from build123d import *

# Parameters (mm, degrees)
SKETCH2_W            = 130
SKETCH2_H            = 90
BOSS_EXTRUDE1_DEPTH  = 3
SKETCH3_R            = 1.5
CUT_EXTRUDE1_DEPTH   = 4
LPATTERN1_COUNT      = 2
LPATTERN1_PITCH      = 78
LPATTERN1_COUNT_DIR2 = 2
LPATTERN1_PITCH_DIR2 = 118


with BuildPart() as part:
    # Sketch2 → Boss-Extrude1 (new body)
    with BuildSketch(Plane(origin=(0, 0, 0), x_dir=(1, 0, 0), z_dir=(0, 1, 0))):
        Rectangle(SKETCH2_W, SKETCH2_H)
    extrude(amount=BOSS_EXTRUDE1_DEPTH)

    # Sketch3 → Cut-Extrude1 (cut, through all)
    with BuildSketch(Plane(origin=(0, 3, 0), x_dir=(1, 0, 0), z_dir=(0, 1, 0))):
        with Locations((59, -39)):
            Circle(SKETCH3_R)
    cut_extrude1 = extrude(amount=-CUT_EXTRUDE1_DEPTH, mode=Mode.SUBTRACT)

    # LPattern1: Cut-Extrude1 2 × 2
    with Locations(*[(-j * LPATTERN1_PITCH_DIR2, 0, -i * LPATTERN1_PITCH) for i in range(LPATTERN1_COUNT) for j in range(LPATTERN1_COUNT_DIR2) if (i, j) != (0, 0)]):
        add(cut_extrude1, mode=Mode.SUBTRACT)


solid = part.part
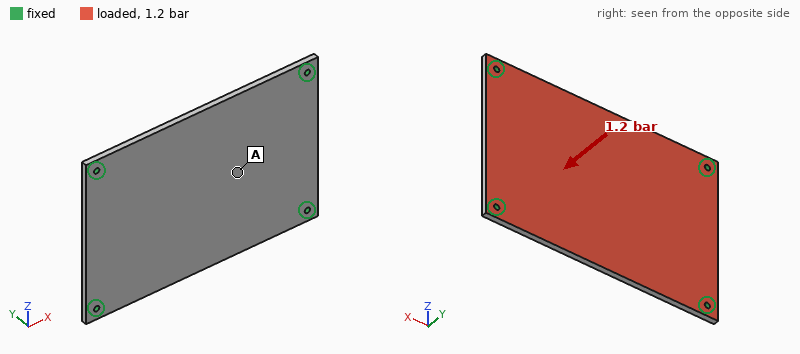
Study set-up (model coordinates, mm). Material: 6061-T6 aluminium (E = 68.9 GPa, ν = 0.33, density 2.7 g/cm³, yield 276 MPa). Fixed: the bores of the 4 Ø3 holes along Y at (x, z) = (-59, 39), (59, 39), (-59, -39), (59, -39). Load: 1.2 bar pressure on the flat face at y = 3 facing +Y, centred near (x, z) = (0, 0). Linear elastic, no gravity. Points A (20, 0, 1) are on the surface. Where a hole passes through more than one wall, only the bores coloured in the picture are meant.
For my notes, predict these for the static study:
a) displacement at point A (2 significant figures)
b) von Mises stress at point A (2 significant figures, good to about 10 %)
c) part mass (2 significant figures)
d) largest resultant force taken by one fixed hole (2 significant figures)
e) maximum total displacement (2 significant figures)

0.59 mm
42 MPa
95 g
350 N
0.68 mm
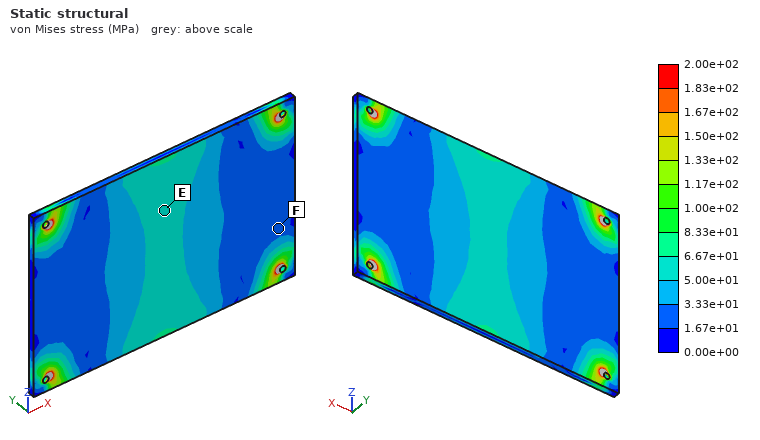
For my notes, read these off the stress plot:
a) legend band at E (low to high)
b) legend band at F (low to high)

5.00e+01 to 6.67e+01 MPa
1.67e+01 to 3.33e+01 MPa
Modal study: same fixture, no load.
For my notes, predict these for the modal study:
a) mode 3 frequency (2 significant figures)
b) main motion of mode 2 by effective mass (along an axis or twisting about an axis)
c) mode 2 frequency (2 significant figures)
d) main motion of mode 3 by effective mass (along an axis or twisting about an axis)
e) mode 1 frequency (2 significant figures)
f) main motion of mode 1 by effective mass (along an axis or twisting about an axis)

2100 Hz
twisting about X
1400 Hz
twisting about Z
860 Hz
along Y
